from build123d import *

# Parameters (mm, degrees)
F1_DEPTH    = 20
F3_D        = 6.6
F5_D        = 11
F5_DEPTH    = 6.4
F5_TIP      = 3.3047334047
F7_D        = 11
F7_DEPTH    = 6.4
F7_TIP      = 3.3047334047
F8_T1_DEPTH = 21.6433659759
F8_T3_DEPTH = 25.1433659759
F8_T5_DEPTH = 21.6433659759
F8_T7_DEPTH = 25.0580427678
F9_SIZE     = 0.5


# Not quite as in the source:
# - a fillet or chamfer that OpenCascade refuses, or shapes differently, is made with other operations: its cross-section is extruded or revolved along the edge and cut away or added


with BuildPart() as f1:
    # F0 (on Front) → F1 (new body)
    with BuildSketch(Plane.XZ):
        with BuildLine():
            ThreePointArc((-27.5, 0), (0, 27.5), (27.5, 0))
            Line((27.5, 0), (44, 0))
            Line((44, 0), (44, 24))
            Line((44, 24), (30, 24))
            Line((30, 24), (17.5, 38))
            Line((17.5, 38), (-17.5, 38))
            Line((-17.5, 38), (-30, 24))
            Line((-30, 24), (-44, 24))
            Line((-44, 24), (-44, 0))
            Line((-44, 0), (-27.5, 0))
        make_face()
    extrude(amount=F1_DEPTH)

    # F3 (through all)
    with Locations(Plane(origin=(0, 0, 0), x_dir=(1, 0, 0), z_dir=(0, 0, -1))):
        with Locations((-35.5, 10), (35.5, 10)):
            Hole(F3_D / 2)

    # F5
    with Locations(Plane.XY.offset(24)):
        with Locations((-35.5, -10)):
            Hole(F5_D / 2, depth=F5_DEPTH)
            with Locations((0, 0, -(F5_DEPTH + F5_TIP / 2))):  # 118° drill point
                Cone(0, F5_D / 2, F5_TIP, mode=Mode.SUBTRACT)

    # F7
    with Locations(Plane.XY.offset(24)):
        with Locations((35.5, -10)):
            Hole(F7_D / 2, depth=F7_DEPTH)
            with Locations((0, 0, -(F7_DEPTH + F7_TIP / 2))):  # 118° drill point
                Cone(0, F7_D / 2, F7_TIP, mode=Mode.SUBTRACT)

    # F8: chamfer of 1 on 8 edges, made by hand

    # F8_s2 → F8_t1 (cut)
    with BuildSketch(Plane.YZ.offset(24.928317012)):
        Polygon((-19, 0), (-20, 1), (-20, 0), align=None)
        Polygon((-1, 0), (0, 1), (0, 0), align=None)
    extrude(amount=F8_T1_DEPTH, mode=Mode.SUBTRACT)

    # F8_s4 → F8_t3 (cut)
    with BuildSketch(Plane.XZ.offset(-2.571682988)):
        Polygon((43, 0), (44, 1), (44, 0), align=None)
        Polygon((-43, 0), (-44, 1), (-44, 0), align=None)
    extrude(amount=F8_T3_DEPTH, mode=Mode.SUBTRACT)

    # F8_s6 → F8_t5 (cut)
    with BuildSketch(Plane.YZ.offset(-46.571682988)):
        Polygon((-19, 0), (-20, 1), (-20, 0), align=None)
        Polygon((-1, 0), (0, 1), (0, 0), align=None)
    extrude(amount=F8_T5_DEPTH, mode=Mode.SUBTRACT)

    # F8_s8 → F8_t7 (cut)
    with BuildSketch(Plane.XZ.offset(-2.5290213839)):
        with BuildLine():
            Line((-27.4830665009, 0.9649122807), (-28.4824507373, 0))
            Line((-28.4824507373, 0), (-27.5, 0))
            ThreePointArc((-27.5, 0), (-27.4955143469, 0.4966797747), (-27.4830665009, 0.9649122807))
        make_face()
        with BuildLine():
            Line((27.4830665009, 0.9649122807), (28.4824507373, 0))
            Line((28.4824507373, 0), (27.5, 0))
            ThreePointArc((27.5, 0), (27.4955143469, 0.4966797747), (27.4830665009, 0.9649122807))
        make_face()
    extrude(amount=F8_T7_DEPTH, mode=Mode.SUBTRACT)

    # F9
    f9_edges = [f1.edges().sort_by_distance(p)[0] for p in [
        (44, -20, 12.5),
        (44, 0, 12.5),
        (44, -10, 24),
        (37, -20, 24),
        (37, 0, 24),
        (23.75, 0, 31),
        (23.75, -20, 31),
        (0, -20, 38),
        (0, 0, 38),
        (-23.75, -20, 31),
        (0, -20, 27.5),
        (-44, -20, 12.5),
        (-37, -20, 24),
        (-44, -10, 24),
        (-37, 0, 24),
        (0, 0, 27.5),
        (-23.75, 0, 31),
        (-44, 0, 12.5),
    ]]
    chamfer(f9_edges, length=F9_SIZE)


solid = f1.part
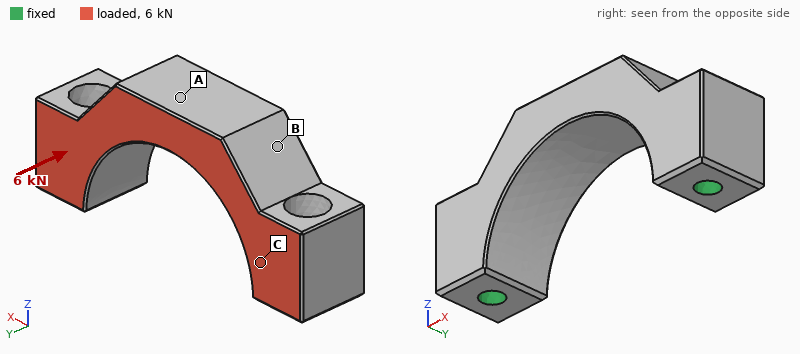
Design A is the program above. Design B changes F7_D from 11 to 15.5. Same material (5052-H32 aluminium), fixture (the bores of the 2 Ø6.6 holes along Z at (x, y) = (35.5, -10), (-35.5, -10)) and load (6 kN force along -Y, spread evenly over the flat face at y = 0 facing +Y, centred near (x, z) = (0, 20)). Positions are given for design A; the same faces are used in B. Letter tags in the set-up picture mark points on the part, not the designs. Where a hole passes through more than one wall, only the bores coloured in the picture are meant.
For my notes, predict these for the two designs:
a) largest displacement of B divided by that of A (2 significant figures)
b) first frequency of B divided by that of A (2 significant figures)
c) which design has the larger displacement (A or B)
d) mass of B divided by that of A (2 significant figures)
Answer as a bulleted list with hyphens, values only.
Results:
- 1.1
- 0.96
- B
- 0.98
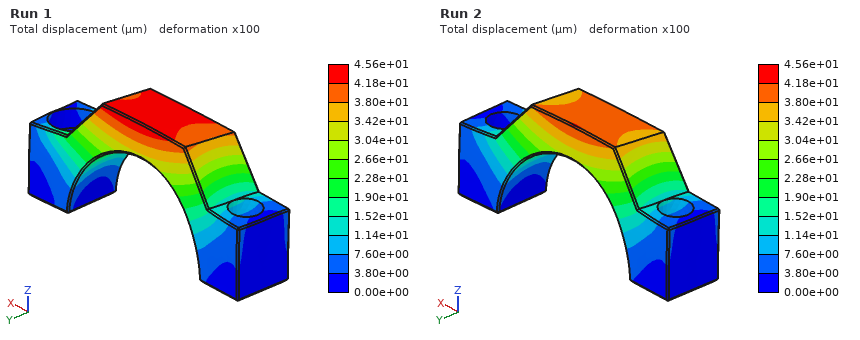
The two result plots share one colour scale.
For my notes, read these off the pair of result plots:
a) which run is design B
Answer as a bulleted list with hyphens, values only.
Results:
- Run 1
